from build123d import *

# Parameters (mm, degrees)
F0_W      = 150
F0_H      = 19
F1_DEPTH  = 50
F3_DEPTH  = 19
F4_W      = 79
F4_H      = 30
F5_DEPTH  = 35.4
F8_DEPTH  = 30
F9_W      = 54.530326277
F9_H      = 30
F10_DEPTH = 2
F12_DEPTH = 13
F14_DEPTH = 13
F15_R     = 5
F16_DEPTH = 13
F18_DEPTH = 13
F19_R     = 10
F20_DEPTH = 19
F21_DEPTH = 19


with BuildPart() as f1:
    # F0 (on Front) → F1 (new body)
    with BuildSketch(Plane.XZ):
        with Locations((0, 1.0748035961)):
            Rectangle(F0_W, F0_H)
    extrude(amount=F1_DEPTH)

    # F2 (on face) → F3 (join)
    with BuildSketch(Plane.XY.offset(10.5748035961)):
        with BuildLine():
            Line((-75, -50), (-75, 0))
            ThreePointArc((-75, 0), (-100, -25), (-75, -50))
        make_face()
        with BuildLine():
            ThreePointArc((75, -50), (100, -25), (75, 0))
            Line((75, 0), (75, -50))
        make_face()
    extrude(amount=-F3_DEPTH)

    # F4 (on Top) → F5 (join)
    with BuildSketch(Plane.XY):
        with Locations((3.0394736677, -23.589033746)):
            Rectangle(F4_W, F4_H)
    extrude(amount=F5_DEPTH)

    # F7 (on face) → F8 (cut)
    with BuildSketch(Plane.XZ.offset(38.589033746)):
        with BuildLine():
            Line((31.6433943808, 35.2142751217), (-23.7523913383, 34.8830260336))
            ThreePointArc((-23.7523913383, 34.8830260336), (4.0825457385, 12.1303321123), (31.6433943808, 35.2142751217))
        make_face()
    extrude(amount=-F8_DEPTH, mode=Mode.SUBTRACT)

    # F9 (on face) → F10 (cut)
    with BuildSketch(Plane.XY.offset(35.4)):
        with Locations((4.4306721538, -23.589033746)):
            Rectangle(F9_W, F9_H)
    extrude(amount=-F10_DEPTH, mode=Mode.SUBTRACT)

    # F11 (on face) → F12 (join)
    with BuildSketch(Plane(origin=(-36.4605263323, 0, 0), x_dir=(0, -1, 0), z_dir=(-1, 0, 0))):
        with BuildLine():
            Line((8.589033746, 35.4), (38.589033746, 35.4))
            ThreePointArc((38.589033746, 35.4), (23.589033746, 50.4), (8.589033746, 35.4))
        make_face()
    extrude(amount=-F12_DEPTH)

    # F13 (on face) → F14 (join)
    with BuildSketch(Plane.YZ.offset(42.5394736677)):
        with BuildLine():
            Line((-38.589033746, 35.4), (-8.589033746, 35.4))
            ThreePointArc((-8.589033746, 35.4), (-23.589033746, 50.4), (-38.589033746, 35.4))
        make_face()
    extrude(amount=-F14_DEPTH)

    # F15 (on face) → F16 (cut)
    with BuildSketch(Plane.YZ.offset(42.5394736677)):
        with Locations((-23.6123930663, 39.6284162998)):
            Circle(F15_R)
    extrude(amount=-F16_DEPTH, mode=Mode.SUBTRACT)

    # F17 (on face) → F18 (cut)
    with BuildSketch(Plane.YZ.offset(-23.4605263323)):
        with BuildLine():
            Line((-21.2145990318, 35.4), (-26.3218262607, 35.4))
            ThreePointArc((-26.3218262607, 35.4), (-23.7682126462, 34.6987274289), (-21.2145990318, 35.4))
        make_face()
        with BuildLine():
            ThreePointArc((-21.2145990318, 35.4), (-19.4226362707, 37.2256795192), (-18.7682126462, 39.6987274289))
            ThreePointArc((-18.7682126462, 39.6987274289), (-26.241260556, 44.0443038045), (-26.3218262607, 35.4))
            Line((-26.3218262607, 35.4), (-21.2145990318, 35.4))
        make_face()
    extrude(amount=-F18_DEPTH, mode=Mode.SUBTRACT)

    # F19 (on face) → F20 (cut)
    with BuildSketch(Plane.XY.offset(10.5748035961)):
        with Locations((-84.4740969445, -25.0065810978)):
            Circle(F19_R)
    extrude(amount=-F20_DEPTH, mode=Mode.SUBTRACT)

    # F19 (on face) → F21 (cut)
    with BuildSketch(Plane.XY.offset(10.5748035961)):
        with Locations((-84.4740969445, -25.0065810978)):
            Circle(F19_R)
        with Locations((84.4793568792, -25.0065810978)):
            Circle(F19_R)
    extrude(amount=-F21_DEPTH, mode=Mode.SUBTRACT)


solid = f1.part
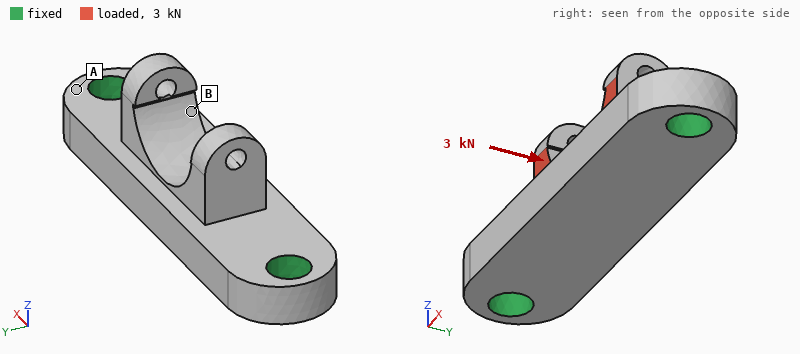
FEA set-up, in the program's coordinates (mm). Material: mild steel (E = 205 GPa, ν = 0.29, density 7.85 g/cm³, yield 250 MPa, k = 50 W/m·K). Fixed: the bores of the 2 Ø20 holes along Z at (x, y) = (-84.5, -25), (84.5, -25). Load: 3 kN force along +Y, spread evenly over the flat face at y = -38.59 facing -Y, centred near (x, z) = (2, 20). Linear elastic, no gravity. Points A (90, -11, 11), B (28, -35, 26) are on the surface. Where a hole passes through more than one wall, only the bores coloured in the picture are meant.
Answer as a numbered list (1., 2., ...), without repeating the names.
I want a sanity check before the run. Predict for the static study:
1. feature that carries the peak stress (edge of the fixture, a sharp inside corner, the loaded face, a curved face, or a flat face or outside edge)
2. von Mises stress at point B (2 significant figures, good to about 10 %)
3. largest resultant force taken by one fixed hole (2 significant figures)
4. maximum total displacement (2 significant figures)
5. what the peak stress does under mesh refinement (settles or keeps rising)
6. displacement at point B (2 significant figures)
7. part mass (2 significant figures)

1. edge of the fixture
2. 3.4 MPa
3. 1.5 kN
4. 12 µm
5. keeps rising
6. 7.3 µm
7. 1.6 kg
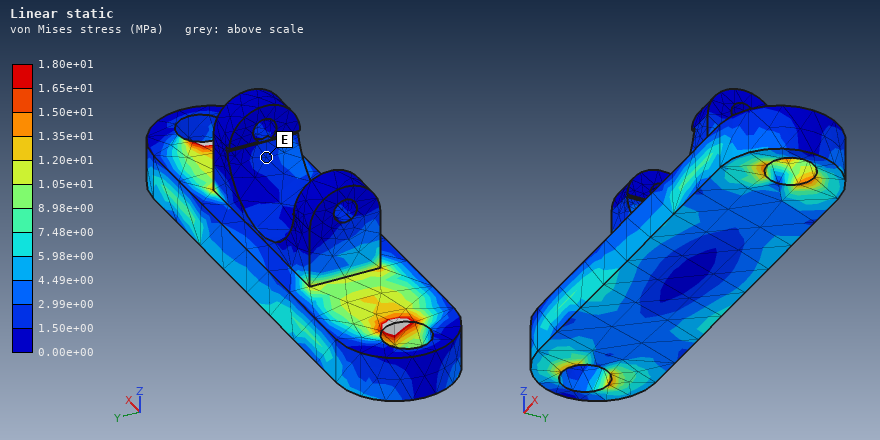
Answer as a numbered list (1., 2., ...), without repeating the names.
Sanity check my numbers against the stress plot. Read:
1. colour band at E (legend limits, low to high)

1. 1.50e+00 to 2.99e+00 MPa
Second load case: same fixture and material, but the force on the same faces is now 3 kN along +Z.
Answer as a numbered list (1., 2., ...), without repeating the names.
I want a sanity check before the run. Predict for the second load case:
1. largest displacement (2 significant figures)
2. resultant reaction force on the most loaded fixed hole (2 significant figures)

1. 11 µm
2. 1.6 kN
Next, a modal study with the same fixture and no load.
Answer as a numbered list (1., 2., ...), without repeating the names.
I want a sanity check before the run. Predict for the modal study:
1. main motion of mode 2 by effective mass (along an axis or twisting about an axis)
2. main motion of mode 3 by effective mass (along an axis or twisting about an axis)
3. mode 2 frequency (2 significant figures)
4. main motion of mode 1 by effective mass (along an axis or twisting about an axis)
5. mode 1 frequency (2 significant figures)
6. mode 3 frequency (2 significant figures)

1. along Y
2. along Y
3. 4200 Hz
4. along Z
5. 3300 Hz
6. 5900 Hz
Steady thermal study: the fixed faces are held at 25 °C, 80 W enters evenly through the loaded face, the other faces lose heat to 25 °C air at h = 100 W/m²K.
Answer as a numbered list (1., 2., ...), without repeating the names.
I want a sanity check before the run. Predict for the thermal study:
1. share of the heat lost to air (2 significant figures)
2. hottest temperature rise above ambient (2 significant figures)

1. 57 %
2. 43 K
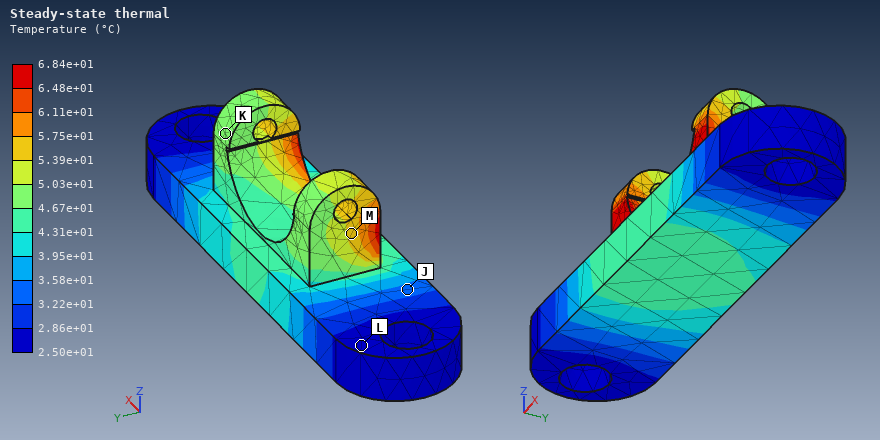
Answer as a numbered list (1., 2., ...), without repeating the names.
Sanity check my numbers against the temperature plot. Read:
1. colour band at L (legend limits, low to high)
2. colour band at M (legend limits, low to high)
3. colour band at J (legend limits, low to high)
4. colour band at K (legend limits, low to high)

1. 2.50e+01 to 2.86e+01 °C
2. 5.39e+01 to 5.75e+01 °C
3. 3.22e+01 to 3.58e+01 °C
4. 4.67e+01 to 5.03e+01 °C
